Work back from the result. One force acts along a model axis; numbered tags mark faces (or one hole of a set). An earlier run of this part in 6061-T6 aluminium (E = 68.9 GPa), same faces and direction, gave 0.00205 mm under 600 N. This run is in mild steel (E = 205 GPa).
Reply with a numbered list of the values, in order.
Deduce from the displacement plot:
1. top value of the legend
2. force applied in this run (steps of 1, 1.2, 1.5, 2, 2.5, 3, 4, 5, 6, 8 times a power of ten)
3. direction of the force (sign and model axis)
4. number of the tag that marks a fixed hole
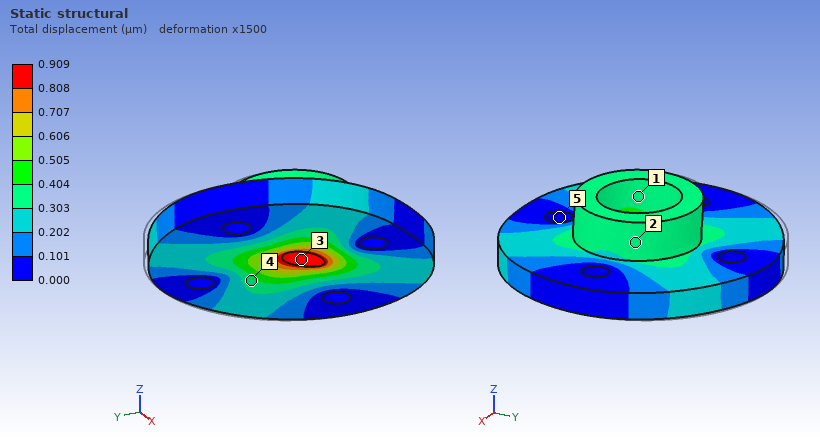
1. 0.909 µm
2. 800 N
3. -Y
4. 5
